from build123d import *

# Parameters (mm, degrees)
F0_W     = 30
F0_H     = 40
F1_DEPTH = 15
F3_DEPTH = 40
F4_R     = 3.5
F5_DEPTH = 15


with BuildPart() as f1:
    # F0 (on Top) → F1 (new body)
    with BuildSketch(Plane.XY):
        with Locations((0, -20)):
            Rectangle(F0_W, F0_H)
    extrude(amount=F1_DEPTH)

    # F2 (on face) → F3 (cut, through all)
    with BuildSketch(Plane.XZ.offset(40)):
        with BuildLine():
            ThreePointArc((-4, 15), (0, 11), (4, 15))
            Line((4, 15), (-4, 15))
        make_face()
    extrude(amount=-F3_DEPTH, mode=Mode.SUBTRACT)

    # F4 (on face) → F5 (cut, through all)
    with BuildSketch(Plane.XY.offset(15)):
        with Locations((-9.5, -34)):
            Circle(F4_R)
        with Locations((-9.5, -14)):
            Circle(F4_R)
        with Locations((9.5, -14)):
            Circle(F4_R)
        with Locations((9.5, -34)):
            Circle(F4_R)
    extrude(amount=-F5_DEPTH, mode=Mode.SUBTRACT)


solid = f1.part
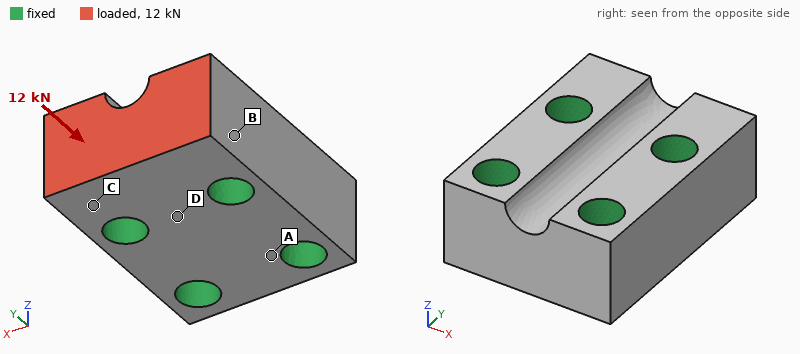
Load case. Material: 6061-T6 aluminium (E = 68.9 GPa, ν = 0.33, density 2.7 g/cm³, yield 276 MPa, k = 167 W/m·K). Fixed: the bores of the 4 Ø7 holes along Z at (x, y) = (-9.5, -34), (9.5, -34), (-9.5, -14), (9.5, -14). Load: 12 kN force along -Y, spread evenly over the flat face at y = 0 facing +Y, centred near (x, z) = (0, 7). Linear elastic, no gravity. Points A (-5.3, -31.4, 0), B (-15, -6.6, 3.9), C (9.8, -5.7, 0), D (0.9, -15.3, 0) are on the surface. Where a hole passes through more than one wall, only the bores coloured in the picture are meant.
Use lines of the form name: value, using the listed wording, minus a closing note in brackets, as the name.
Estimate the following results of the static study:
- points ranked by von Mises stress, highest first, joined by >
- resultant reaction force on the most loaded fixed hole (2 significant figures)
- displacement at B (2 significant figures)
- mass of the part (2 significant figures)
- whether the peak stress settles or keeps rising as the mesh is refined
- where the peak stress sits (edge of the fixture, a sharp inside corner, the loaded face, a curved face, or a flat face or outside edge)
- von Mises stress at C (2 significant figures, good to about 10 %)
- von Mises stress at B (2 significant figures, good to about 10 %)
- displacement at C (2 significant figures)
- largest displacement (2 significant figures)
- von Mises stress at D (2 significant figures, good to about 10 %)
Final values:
points ranked by von Mises stress, highest first, joined by >: C > B > D > A
resultant reaction force on the most loaded fixed hole: 5.8 kN
displacement at B: 3.0 µm
mass of the part: 40 g
whether the peak stress settles or keeps rising as the mesh is refined: keeps rising
where the peak stress sits: edge of the fixture
von Mises stress at C: 31 MPa
von Mises stress at B: 23 MPa
displacement at C: 3.0 µm
largest displacement: 5.7 µm
von Mises stress at D: 12 MPa
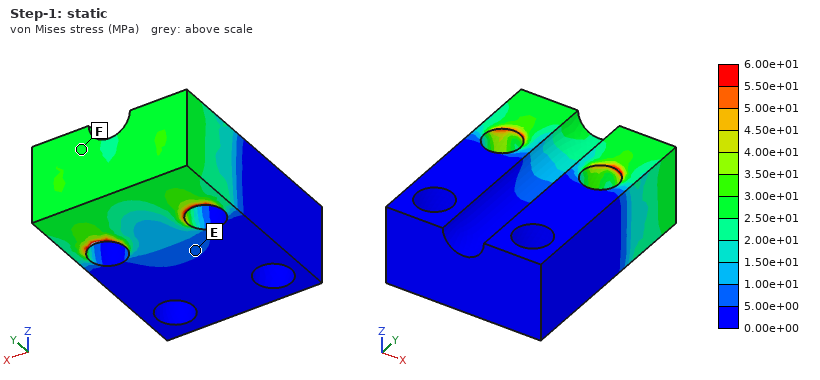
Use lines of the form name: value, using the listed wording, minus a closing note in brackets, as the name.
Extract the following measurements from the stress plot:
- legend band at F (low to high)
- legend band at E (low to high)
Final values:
legend band at F: 2.50e+01 to 3.00e+01 MPa
legend band at E: 5.00e+00 to 1.00e+01 MPa
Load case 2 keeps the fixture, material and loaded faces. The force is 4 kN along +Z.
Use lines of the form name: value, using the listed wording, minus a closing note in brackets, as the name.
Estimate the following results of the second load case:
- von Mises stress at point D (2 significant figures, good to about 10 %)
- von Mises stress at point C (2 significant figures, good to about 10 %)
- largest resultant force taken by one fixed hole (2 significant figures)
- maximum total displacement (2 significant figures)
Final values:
von Mises stress at point D: 15 MPa
von Mises stress at point C: 27 MPa
largest resultant force taken by one fixed hole: 2.1 kN
maximum total displacement: 12 µm
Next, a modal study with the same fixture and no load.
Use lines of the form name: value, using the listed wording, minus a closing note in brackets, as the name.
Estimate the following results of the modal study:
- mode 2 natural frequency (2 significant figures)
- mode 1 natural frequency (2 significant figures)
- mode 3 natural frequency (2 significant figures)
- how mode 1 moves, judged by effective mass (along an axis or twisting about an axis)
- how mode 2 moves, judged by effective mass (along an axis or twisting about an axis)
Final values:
mode 2 natural frequency: 53 kHz
mode 1 natural frequency: 47 kHz
mode 3 natural frequency: 57 kHz
how mode 1 moves, judged by effective mass: along Z
how mode 2 moves, judged by effective mass: along X
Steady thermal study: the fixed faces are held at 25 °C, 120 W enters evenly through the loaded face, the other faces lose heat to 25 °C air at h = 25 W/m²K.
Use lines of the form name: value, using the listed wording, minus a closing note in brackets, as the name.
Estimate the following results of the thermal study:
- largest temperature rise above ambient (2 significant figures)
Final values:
largest temperature rise above ambient: 21 K
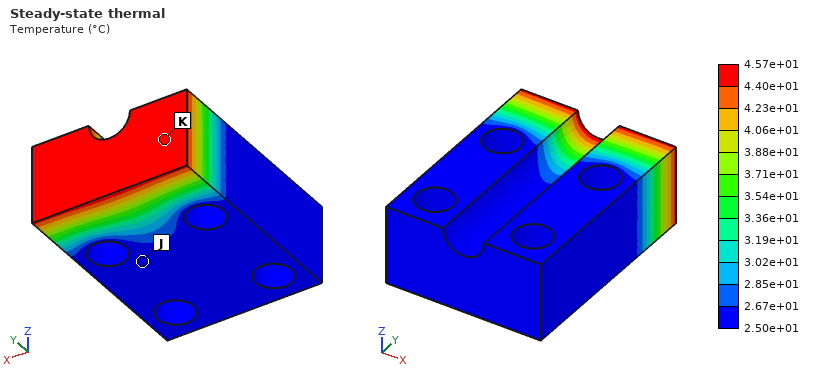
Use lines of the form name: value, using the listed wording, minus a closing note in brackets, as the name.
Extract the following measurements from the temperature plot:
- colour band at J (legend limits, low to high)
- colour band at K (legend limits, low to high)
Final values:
colour band at J: 2.50e+01 to 2.67e+01 °C
colour band at K: 4.40e+01 to 4.57e+01 °C
